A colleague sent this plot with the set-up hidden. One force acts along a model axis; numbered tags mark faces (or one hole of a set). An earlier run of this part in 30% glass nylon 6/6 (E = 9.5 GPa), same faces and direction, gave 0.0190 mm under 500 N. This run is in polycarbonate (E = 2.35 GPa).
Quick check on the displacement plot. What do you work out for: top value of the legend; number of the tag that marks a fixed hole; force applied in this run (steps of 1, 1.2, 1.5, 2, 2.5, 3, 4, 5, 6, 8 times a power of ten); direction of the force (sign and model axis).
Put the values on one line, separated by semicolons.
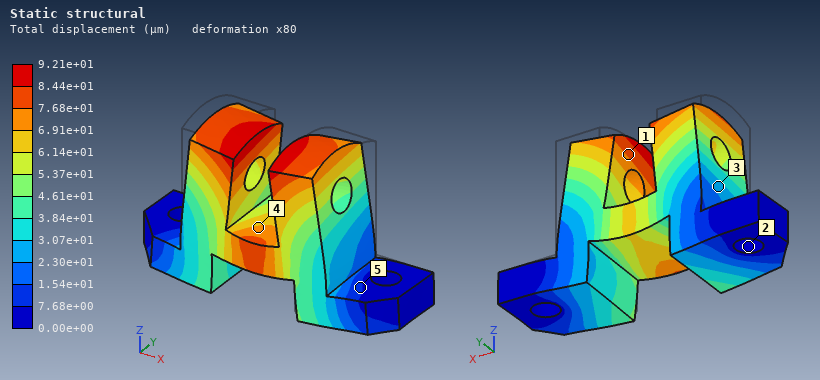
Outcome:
9.21e+01 µm; 2; 600 N; -Z
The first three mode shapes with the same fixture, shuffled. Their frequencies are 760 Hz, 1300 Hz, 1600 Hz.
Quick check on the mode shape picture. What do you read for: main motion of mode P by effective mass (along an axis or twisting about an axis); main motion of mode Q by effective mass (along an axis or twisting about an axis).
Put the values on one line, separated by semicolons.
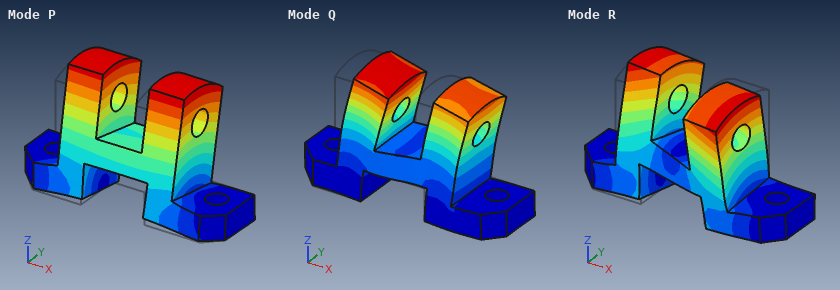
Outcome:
along Y; along X
